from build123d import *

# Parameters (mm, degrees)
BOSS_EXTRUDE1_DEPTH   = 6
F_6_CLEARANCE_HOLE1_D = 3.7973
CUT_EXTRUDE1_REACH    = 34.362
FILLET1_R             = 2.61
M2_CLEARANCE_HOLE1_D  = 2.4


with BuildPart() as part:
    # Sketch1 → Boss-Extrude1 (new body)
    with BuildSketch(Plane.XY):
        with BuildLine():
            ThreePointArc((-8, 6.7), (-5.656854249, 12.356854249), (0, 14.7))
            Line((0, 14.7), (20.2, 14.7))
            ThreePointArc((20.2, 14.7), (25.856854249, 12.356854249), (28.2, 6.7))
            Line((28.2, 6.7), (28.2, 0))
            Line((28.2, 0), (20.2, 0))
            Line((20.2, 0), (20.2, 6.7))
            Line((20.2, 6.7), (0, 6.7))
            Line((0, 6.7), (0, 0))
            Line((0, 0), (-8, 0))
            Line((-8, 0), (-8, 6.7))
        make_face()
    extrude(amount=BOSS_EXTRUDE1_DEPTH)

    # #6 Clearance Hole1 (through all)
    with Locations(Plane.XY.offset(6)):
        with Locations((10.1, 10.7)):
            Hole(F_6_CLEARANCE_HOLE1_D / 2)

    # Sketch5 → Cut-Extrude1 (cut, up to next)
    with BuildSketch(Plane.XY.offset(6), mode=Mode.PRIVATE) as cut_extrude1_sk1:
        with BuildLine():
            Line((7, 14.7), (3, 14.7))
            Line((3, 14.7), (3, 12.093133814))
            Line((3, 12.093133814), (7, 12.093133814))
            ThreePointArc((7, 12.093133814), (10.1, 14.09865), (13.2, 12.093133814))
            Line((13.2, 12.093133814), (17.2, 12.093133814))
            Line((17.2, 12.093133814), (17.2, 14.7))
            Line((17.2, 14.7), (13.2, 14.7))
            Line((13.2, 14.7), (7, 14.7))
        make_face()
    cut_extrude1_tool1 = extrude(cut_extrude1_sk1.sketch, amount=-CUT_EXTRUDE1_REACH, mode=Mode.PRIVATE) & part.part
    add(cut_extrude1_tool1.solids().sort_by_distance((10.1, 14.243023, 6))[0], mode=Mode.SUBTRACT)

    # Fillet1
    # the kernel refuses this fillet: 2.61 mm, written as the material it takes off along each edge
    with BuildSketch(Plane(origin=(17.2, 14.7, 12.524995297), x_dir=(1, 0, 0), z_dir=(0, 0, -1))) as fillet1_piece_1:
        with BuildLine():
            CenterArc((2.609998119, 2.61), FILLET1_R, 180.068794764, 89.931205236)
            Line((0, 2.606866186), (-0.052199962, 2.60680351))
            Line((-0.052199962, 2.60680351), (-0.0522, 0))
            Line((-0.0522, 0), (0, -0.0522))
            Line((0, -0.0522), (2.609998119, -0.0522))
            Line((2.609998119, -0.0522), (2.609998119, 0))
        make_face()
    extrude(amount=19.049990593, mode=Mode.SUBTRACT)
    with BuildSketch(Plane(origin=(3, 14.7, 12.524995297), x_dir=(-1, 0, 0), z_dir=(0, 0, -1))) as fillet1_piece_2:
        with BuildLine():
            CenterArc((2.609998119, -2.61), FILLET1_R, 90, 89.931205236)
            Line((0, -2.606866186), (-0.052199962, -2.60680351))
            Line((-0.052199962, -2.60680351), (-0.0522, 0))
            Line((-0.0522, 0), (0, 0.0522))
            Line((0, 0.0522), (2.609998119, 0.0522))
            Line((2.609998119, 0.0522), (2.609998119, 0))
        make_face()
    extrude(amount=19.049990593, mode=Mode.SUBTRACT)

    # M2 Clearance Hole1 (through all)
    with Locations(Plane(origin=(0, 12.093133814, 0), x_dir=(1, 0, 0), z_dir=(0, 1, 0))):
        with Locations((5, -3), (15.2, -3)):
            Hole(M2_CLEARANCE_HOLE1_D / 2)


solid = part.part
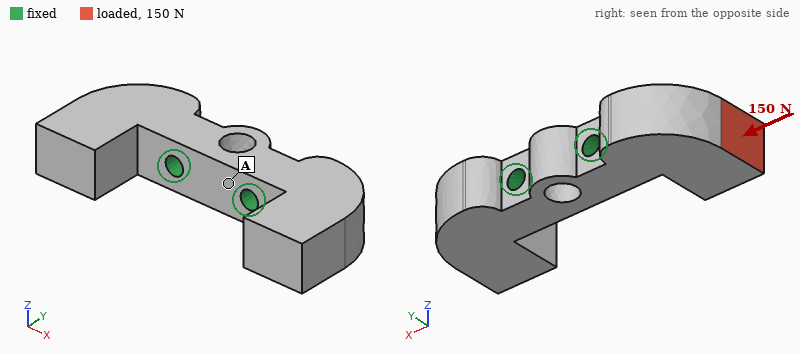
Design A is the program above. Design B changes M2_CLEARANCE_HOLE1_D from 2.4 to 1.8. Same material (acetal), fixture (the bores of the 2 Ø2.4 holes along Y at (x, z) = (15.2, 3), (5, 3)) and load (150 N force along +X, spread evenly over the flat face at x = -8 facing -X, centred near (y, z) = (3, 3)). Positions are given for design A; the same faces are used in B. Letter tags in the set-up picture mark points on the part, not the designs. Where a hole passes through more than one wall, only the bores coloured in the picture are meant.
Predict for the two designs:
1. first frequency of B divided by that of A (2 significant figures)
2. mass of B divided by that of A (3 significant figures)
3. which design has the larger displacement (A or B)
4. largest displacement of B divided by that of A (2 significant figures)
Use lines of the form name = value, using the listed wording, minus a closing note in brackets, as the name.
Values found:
first frequency of B divided by that of A = 0.91
mass of B divided by that of A = 1.01
which design has the larger displacement = B
largest displacement of B divided by that of A = 1.1
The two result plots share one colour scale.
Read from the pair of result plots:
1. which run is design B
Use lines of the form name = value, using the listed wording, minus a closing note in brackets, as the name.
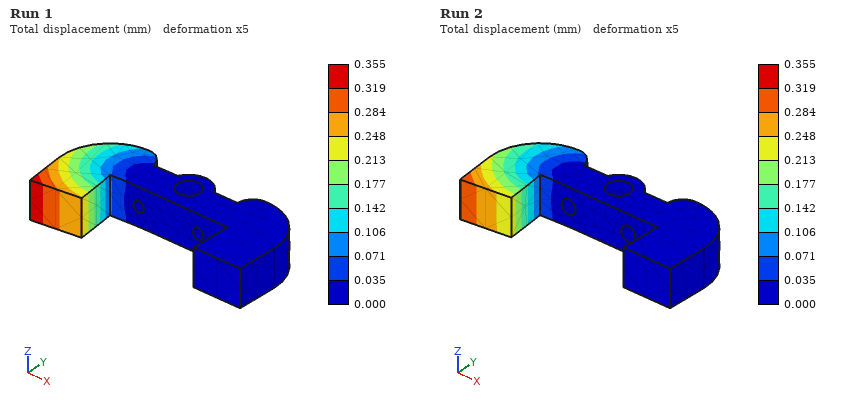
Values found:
which run is design B = Run 1
